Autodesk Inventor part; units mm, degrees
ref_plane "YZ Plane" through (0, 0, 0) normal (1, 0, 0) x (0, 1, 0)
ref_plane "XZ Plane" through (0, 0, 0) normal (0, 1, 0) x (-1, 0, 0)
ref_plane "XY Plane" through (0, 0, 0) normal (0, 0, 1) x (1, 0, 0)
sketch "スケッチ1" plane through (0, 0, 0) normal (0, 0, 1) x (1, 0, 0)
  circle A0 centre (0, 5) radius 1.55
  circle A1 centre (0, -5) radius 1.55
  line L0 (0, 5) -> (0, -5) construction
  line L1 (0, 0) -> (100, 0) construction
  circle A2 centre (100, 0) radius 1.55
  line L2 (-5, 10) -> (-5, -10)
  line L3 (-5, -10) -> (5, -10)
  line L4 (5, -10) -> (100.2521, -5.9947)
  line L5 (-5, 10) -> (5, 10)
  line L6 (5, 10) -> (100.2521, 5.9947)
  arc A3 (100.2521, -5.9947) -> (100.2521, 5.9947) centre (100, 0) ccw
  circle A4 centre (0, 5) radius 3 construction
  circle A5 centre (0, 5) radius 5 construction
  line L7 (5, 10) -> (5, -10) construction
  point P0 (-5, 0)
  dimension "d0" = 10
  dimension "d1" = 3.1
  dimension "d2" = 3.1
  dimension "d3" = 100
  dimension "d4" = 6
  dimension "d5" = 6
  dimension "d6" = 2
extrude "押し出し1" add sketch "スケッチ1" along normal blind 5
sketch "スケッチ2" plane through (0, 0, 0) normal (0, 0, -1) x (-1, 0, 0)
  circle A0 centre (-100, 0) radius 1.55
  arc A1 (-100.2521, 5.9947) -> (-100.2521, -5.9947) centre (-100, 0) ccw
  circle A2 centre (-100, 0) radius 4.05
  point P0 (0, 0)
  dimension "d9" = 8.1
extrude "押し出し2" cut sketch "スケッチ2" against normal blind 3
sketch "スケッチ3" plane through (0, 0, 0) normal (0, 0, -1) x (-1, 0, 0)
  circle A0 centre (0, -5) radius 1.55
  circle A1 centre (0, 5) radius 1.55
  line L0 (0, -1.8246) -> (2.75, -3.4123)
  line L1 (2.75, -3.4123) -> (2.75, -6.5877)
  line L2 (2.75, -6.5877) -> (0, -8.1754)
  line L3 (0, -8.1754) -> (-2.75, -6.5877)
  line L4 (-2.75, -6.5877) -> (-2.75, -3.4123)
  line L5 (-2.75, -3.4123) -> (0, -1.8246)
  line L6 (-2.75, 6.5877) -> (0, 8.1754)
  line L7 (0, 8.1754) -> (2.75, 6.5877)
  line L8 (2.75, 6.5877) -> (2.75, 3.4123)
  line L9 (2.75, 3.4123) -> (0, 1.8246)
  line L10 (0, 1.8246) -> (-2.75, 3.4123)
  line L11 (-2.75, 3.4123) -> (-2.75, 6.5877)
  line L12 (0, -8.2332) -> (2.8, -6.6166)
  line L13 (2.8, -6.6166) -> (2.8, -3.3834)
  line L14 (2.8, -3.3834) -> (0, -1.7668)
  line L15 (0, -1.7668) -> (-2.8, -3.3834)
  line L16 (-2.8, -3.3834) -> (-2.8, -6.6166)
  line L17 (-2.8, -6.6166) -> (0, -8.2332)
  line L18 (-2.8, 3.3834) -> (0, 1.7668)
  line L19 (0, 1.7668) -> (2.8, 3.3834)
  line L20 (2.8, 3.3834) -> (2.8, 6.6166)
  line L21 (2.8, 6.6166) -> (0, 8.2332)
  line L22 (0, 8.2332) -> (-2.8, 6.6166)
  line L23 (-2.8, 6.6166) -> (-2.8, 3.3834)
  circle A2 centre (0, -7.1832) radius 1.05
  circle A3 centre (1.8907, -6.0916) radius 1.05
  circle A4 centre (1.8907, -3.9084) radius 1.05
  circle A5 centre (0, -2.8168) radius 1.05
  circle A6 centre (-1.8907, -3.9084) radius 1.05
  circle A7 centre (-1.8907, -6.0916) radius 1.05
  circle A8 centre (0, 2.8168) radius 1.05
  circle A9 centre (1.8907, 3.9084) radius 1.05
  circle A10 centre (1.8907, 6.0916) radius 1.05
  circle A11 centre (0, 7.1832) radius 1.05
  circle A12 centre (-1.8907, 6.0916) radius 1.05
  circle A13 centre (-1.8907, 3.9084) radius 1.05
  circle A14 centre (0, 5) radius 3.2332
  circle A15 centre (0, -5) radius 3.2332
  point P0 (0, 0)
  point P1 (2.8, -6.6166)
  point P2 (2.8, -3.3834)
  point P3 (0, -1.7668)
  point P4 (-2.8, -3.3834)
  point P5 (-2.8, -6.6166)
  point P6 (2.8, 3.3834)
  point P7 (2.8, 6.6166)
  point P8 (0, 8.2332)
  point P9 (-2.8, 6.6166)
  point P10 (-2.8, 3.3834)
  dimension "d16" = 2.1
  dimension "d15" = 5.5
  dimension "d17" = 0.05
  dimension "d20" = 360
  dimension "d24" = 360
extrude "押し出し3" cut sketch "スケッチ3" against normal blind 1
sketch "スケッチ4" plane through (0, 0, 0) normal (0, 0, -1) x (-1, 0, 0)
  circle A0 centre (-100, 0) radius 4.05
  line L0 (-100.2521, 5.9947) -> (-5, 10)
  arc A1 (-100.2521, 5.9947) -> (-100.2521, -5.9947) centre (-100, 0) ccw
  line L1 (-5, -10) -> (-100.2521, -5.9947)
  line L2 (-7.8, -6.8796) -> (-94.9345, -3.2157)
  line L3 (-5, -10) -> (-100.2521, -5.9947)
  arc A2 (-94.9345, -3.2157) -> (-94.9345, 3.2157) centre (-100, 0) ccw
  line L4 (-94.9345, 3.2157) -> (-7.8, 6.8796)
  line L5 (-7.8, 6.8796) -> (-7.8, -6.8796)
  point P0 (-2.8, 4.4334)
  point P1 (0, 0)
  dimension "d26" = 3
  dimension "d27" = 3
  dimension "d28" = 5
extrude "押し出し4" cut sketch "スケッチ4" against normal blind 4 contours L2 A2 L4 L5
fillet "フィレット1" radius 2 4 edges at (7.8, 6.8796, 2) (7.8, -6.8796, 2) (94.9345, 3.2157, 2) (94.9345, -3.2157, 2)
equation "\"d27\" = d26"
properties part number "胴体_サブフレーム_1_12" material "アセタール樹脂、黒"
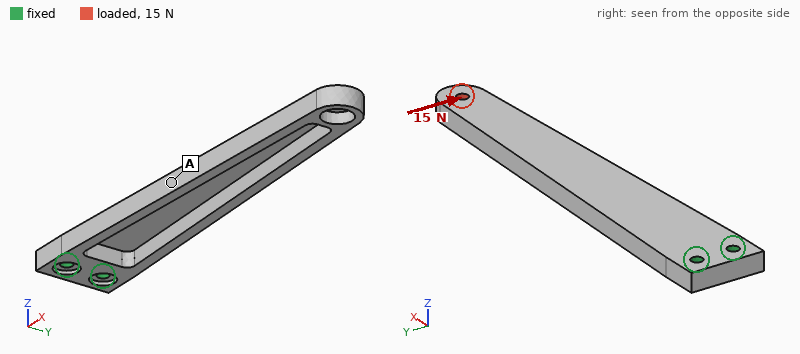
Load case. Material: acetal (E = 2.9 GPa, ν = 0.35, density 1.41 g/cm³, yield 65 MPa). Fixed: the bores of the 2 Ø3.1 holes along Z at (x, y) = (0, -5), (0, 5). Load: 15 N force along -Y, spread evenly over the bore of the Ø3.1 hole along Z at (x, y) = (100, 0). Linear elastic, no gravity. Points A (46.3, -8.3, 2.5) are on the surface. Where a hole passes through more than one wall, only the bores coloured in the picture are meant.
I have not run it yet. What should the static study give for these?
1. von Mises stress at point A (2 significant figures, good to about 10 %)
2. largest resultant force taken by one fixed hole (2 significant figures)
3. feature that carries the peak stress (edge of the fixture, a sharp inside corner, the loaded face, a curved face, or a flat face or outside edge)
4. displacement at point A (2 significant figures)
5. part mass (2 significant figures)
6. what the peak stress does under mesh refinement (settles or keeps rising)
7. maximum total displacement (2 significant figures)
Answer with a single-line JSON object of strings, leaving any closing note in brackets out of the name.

{"von Mises stress at point A": "4.6 MPa", "largest resultant force taken by one fixed hole": "120 N", "feature that carries the peak stress": "edge of the fixture", "displacement at point A": "0.28 mm", "part mass": "7.2 g", "what the peak stress does under mesh refinement": "keeps rising", "maximum total displacement": "1.2 mm"}
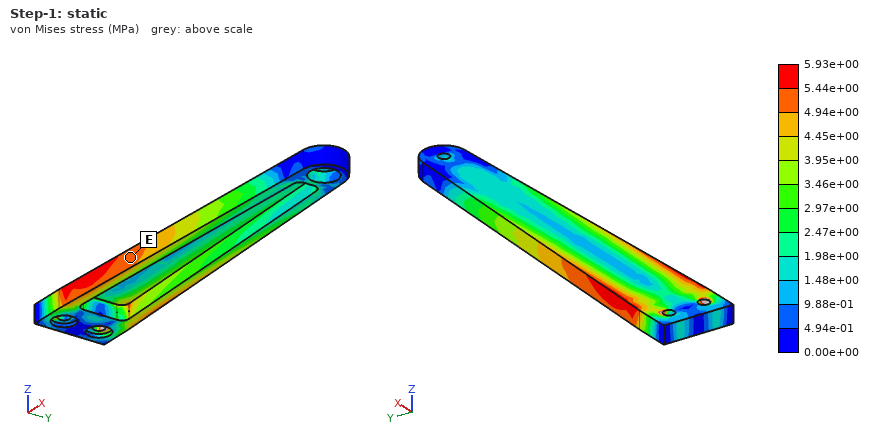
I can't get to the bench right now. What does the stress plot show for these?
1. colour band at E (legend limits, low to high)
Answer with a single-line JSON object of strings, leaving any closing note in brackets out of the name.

{"colour band at E": "4.94e+00 to 5.44e+00 MPa"}
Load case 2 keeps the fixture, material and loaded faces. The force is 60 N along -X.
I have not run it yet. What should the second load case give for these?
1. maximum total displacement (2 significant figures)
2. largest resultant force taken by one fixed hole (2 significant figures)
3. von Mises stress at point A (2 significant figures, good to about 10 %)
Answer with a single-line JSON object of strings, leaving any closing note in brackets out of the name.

{"maximum total displacement": "1.1 mm", "largest resultant force taken by one fixed hole": "30 N", "von Mises stress at point A": "1.2 MPa"}
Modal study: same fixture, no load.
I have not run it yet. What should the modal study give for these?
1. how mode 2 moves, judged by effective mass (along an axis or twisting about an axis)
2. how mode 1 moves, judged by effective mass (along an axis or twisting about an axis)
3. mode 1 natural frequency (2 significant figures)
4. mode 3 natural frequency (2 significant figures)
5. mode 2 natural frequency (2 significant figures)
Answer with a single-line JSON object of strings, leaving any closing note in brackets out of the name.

{"how mode 2 moves, judged by effective mass": "along Y", "how mode 1 moves, judged by effective mass": "along Z", "mode 1 natural frequency": "120 Hz", "mode 3 natural frequency": "680 Hz", "mode 2 natural frequency": "430 Hz"}
